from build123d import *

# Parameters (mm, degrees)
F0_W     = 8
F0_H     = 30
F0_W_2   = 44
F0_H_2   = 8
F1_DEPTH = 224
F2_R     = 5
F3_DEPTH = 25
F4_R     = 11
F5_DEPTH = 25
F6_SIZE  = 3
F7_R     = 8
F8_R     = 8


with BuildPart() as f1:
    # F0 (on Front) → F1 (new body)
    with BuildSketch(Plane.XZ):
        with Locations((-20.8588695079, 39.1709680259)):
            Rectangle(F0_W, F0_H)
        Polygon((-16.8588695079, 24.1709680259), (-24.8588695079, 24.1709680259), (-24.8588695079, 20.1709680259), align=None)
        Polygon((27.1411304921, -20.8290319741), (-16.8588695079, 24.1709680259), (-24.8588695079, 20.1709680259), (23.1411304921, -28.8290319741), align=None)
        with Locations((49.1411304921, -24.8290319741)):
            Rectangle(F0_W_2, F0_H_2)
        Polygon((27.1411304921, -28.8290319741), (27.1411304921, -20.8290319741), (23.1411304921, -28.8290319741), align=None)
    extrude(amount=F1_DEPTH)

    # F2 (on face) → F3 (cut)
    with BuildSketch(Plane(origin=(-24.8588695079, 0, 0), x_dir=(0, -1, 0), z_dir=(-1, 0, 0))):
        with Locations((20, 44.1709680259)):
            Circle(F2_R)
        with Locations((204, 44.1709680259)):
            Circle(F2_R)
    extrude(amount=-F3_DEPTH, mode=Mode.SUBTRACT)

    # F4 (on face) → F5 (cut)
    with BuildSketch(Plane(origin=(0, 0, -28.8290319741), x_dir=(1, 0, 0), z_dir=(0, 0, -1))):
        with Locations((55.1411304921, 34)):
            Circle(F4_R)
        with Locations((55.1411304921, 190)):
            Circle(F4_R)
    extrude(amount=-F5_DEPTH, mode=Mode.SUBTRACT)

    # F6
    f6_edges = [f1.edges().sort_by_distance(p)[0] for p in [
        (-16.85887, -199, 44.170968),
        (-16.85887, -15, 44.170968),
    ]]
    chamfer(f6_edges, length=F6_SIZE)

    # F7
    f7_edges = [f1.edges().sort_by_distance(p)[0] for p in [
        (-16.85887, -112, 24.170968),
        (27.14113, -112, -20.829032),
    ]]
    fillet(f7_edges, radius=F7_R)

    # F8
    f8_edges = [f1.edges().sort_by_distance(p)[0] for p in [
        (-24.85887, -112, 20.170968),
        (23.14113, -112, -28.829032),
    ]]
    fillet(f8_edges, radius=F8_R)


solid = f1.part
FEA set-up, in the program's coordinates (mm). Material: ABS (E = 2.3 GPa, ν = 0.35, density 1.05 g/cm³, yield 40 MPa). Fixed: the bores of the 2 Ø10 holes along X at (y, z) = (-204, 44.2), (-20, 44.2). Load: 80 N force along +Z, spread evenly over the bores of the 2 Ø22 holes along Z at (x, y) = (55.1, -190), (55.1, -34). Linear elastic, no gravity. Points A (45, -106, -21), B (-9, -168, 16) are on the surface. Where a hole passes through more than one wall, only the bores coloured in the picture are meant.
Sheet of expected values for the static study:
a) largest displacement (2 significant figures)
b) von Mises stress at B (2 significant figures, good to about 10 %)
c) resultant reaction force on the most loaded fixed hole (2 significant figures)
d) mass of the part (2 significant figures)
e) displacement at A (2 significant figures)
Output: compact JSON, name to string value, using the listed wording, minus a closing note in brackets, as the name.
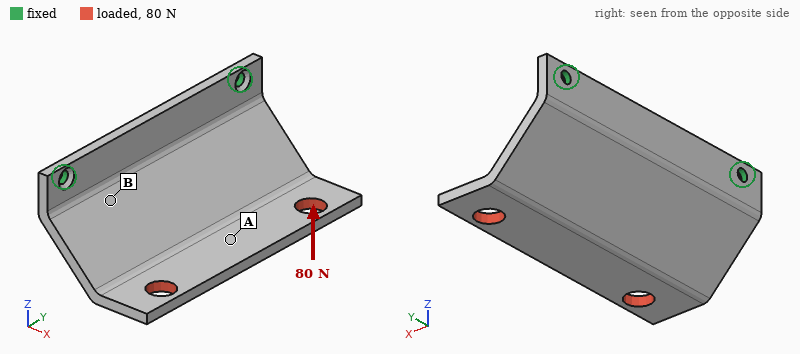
{"largest displacement": "2.7 mm", "von Mises stress at B": "1.9 MPa", "resultant reaction force on the most loaded fixed hole": "56 N", "mass of the part": "270 g", "displacement at A": "1.9 mm"}
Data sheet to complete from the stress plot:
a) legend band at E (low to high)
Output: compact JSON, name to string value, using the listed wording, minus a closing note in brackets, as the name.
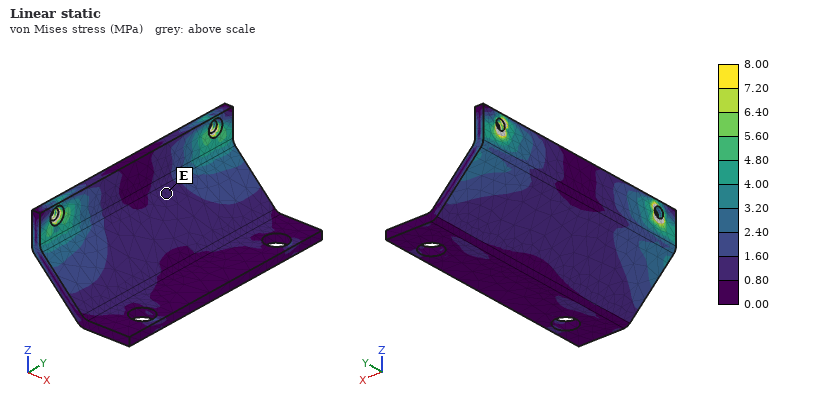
{"legend band at E": "0.80 to 1.60 MPa"}
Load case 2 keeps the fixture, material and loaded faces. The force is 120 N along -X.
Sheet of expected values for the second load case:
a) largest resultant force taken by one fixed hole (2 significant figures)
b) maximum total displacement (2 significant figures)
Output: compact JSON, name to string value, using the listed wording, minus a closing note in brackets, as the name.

{"largest resultant force taken by one fixed hole": "67 N", "maximum total displacement": "2.7 mm"}
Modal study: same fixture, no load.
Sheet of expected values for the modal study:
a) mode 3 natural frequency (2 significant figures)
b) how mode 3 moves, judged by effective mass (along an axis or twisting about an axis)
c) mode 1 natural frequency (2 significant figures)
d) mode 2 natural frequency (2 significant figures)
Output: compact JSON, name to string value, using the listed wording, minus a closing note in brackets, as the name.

{"mode 3 natural frequency": "430 Hz", "how mode 3 moves, judged by effective mass": "along X", "mode 1 natural frequency": "89 Hz", "mode 2 natural frequency": "200 Hz"}
